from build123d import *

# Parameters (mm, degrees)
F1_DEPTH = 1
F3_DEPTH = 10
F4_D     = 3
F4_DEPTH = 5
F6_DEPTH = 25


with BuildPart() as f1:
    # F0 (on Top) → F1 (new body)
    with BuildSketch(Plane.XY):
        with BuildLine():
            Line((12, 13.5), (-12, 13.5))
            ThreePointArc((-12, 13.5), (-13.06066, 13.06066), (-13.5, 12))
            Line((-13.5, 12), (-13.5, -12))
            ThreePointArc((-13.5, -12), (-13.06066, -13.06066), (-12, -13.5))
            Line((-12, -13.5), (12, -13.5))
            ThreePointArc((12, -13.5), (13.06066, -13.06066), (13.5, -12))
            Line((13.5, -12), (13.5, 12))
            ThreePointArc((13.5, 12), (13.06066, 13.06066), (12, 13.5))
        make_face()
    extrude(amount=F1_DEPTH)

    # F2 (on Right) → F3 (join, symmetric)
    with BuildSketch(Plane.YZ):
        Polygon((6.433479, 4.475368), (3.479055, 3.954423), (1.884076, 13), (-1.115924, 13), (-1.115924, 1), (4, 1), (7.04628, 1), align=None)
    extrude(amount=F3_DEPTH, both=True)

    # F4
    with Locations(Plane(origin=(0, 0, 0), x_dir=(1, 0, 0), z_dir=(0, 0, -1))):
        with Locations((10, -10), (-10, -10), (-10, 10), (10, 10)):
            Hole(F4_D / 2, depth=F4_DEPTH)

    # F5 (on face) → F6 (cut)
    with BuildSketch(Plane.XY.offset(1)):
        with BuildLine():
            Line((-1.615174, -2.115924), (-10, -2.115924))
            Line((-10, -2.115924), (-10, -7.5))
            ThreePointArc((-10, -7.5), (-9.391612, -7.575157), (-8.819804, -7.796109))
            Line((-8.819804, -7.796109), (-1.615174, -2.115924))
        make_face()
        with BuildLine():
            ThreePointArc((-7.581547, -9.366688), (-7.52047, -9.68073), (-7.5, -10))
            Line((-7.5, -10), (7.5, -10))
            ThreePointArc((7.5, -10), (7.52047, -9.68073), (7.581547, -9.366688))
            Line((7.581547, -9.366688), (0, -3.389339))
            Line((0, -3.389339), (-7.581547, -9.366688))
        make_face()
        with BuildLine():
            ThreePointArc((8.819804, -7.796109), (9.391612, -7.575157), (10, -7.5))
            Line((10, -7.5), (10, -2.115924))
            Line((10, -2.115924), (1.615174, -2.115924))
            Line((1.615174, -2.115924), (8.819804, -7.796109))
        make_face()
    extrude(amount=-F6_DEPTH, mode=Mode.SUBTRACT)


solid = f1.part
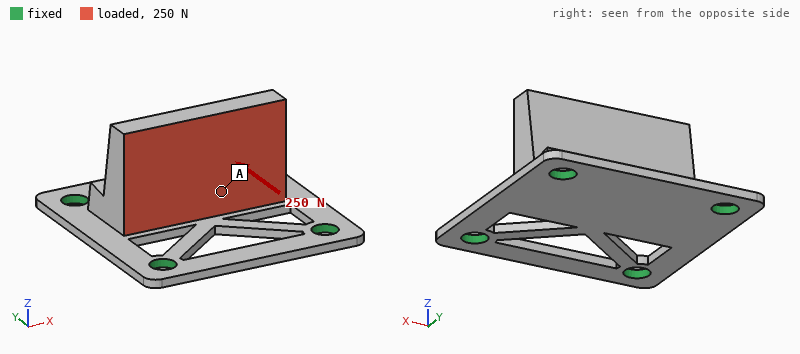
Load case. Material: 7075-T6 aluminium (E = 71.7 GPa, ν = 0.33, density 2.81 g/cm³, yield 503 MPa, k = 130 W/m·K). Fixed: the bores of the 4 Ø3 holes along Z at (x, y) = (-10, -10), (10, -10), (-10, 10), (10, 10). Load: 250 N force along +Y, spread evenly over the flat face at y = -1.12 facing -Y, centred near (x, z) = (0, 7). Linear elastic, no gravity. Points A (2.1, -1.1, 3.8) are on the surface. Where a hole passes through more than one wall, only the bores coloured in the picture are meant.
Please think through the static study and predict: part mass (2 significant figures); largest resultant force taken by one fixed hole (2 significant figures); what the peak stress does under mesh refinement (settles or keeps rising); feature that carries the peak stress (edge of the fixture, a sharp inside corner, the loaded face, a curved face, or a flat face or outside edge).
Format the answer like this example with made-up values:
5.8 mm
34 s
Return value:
4.9 g
120 N
keeps rising
a sharp inside corner
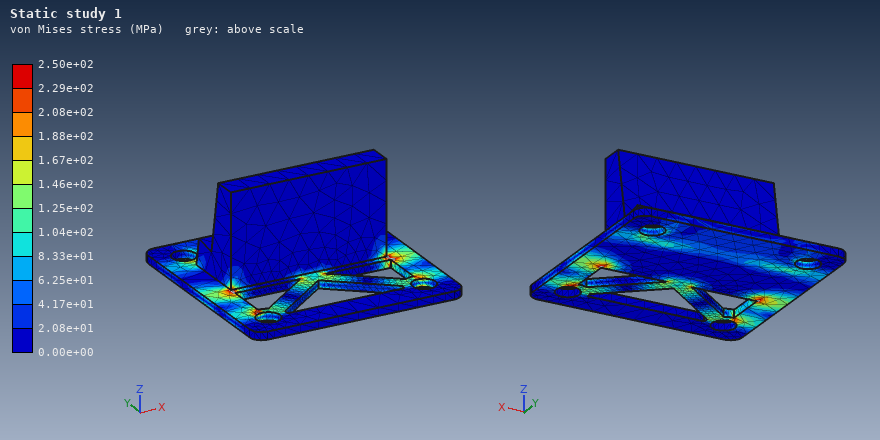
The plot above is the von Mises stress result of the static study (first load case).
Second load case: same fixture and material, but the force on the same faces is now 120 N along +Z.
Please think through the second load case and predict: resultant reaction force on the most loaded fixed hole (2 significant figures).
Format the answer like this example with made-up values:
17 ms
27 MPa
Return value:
31 N
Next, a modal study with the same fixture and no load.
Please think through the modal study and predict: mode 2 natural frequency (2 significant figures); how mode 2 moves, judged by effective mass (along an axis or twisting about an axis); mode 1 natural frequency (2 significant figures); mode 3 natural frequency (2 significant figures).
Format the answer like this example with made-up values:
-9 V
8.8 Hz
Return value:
12 kHz
along X
4100 Hz
16 kHz
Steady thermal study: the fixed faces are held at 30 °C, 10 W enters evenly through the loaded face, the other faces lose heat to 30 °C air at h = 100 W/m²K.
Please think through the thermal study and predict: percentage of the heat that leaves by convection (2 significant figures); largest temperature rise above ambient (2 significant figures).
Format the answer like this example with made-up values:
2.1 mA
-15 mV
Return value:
15 %
19 K
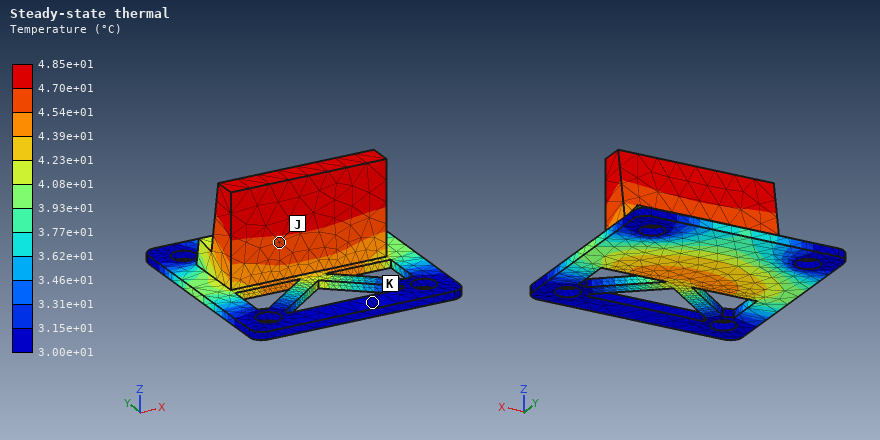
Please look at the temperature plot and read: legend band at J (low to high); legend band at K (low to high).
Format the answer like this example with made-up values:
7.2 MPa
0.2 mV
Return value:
4.54e+01 to 4.70e+01 °C
3.00e+01 to 3.15e+01 °C
